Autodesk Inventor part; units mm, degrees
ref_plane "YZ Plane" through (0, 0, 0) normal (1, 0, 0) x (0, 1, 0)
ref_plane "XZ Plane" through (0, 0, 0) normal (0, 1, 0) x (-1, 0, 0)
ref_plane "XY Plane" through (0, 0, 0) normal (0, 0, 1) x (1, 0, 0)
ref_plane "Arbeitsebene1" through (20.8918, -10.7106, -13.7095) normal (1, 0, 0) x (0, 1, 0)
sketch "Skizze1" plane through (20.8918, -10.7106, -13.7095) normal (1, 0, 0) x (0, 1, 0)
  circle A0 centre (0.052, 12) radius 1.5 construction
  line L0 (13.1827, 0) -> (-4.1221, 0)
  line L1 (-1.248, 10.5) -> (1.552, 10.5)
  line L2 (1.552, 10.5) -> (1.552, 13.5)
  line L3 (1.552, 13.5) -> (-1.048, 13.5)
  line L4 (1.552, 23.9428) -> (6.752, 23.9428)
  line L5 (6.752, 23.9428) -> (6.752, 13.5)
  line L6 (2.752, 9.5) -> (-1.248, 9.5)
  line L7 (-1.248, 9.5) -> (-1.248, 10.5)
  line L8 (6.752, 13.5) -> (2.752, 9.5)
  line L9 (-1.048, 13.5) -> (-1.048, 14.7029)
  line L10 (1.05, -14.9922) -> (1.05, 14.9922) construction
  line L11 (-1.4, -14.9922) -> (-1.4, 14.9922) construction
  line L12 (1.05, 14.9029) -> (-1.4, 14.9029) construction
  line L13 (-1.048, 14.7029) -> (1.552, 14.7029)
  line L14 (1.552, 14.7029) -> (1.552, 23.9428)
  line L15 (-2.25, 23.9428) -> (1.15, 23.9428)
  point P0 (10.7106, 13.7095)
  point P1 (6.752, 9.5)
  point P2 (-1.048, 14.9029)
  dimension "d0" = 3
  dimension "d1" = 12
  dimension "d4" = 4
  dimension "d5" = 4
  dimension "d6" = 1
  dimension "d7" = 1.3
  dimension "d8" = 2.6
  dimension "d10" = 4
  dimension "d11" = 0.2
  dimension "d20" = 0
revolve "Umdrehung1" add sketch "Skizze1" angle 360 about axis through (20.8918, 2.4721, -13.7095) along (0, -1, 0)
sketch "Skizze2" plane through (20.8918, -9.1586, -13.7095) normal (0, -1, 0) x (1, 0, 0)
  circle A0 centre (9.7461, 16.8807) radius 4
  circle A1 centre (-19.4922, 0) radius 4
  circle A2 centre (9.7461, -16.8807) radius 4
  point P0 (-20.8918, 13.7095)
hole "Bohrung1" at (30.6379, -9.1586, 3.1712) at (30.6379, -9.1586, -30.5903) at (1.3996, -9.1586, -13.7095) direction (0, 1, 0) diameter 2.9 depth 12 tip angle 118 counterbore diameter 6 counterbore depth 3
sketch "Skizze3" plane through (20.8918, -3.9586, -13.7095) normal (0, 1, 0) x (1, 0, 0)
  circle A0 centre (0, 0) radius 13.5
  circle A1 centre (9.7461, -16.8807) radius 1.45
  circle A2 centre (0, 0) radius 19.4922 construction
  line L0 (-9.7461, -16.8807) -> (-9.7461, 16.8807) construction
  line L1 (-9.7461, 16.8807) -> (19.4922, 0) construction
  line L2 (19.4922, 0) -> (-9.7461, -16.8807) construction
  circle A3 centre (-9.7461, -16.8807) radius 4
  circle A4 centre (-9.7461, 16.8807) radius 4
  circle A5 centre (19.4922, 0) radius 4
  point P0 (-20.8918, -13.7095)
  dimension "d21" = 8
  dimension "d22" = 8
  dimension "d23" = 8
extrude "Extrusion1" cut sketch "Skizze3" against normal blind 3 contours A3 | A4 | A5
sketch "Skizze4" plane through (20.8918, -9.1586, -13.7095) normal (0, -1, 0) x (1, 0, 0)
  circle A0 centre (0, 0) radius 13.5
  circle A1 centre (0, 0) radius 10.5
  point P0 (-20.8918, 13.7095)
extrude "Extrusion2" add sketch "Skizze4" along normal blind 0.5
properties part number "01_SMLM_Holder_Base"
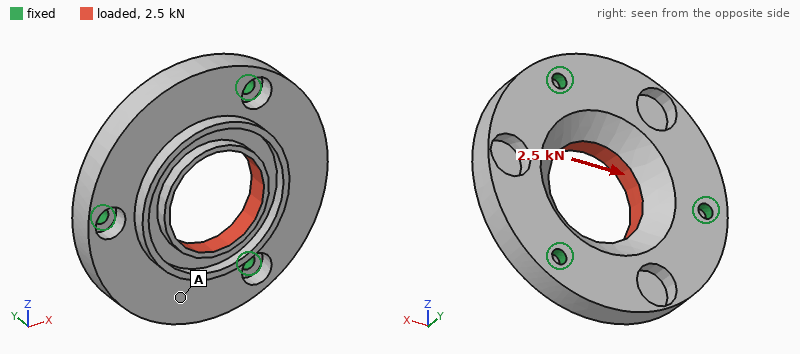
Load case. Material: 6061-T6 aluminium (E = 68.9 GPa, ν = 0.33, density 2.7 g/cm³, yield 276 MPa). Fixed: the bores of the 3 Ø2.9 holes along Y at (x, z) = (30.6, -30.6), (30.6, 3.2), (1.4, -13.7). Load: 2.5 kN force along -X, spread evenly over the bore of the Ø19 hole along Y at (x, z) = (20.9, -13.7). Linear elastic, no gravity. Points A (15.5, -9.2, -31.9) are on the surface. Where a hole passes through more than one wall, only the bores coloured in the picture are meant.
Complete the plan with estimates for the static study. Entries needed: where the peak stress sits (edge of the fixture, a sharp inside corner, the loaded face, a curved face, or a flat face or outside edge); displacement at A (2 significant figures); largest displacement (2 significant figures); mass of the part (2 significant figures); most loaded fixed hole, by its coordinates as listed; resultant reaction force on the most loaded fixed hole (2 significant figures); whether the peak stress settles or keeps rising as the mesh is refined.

edge of the fixture
13 µm
34 µm
19 g
(1.4, -13.7)
970 N
keeps rising
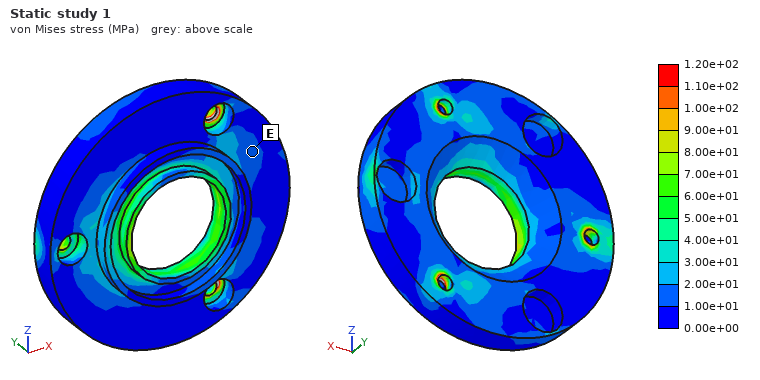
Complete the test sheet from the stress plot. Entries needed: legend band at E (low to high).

1.00e+01 to 2.00e+01 MPa
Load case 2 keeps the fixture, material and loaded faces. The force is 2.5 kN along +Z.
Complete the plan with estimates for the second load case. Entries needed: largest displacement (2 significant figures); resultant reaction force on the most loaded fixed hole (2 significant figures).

29 µm
920 N
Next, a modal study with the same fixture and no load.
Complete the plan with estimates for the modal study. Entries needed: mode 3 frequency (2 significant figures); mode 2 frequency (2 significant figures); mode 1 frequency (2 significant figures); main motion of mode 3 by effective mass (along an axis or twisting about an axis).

14 kHz
10 kHz
10 kHz
along Y
